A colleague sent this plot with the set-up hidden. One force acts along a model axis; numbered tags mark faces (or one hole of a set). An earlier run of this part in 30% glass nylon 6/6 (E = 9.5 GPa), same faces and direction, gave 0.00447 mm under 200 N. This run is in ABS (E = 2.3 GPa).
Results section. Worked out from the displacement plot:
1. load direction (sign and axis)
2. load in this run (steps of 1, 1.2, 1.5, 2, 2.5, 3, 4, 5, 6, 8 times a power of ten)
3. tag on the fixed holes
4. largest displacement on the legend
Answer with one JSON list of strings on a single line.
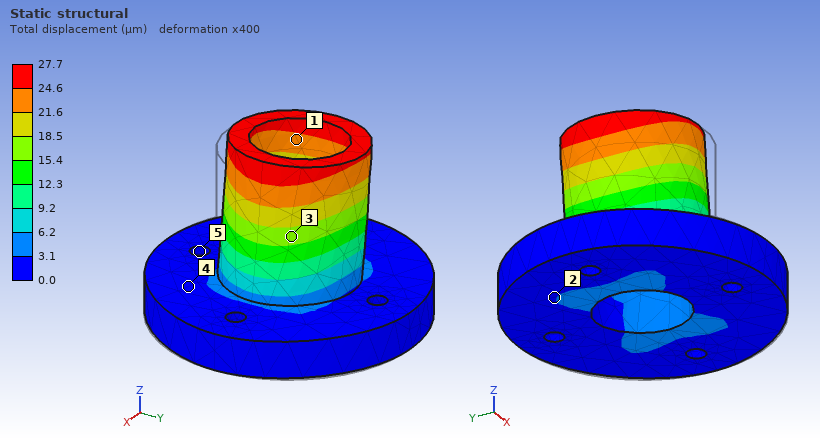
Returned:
["-X", "300 N", "5", "27.7 µm"]
